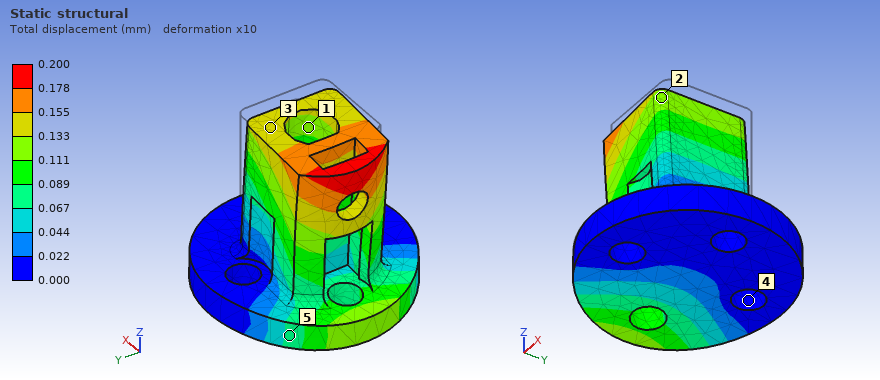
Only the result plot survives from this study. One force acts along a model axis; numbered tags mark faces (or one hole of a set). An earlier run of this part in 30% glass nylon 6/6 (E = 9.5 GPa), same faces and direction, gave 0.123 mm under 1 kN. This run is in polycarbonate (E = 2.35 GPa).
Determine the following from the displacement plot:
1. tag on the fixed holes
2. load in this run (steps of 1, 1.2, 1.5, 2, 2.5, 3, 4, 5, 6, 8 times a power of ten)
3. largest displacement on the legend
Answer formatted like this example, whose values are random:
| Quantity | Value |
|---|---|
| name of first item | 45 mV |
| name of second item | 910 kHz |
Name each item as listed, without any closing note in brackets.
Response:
| Quantity | Value |
|---|---|
| tag on the fixed holes | 4 |
| load in this run | 400 N |
| largest displacement on the legend | 0.200 mm |
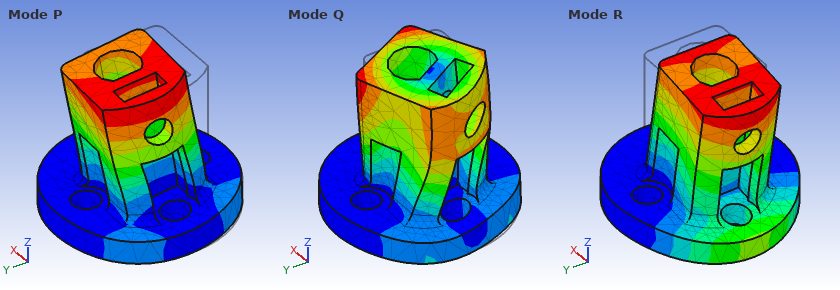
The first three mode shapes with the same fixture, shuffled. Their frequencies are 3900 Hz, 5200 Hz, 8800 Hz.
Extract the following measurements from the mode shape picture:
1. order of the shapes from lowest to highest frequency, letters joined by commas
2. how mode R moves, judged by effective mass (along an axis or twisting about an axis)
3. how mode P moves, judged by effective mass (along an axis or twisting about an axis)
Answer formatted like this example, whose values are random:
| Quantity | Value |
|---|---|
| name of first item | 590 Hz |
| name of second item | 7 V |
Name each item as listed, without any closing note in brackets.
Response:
| Quantity | Value |
|---|---|
| order of the shapes from lowest to highest frequency, letters joined by commas | R, P, Q |
| how mode R moves, judged by effective mass | along X |
| how mode P moves, judged by effective mass | along Y |
